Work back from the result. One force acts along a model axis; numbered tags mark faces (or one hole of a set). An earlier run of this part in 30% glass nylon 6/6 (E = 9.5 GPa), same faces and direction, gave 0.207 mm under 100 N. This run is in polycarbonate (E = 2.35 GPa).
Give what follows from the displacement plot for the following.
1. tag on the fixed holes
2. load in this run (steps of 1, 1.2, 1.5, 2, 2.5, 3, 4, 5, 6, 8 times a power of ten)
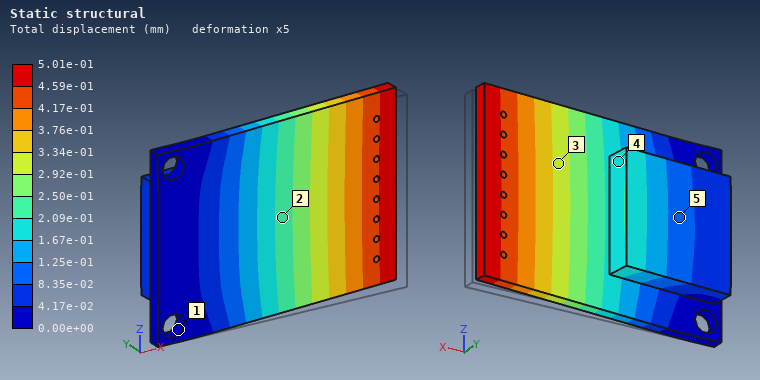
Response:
1
60 N
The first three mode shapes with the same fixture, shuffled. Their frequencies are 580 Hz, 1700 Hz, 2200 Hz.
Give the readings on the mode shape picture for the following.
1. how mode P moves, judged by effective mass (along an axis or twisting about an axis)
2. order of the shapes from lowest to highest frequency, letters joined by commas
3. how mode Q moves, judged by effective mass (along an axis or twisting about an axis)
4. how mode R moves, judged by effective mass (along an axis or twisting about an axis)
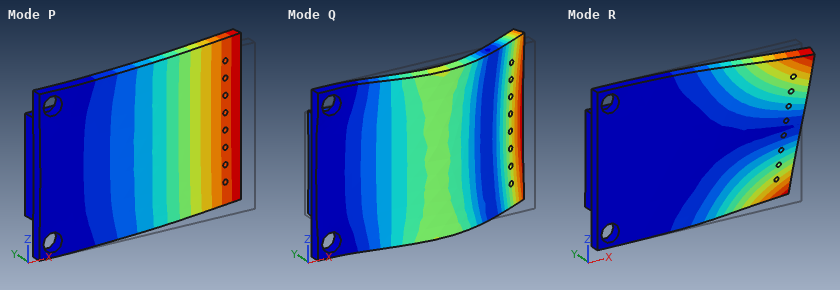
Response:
along Y
P, R, Q
along Y
twisting about X
